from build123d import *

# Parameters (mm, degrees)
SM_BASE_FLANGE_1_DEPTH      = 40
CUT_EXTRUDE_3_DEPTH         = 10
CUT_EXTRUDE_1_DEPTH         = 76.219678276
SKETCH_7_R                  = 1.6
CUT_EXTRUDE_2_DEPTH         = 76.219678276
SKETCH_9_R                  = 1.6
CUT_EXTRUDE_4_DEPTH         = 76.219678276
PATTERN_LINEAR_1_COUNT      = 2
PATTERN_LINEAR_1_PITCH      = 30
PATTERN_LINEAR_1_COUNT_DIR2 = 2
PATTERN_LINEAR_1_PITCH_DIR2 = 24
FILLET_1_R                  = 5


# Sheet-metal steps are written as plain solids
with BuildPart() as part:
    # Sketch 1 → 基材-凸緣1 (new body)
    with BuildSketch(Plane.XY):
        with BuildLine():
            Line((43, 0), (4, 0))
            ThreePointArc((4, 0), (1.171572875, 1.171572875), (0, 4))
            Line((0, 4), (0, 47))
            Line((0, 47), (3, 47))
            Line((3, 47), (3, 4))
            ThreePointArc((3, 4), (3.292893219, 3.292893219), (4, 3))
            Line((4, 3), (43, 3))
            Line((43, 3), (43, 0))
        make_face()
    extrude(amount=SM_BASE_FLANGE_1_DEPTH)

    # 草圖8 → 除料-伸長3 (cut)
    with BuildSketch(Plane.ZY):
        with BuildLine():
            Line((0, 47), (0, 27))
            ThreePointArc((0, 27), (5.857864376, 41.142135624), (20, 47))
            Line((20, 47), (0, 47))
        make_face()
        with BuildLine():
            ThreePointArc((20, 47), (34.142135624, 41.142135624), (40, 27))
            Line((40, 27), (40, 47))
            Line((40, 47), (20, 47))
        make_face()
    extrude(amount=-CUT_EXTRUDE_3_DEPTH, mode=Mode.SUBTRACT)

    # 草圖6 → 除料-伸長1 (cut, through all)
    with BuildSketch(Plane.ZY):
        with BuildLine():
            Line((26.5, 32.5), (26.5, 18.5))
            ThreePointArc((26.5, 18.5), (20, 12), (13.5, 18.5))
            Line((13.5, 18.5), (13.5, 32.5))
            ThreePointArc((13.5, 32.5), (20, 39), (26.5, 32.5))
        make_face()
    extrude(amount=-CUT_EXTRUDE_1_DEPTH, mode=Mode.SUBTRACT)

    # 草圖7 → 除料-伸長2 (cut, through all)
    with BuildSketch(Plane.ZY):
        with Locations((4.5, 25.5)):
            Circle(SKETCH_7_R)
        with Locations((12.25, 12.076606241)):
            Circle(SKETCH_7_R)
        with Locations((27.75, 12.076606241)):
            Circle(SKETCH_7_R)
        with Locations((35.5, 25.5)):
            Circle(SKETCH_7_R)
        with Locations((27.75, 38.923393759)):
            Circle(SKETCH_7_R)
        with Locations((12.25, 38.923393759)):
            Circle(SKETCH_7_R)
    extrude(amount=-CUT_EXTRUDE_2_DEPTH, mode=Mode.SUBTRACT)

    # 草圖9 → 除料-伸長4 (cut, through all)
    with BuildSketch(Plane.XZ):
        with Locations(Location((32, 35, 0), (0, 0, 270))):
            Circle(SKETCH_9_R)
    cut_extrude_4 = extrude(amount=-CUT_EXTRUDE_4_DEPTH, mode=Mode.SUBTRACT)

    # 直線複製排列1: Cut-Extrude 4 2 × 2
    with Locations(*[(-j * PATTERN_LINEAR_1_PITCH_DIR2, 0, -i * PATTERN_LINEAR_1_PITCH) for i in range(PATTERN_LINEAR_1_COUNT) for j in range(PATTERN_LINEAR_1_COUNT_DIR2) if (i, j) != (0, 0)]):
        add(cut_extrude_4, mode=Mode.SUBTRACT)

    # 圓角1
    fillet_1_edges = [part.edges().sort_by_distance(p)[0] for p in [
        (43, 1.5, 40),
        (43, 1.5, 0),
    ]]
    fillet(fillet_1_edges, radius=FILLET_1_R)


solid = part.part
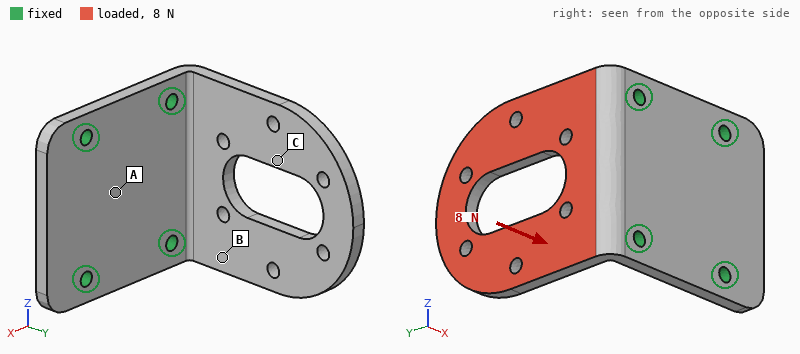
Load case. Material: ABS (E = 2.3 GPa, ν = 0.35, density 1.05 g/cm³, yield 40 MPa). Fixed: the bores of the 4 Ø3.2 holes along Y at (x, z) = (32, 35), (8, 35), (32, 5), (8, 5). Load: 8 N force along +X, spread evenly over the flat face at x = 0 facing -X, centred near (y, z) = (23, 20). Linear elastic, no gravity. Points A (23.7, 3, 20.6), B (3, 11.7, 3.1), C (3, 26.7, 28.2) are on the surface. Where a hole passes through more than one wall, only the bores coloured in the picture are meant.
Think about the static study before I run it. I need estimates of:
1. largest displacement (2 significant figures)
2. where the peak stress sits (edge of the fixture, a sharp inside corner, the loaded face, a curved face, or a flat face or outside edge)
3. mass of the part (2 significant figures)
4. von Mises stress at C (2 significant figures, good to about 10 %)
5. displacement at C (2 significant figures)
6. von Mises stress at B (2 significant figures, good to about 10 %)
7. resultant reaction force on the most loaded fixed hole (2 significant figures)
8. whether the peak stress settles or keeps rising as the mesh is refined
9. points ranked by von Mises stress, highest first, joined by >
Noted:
0.72 mm
edge of the fixture
9.0 g
0.97 MPa
0.32 mm
2.0 MPa
3.0 N
keeps rising
B > C > A
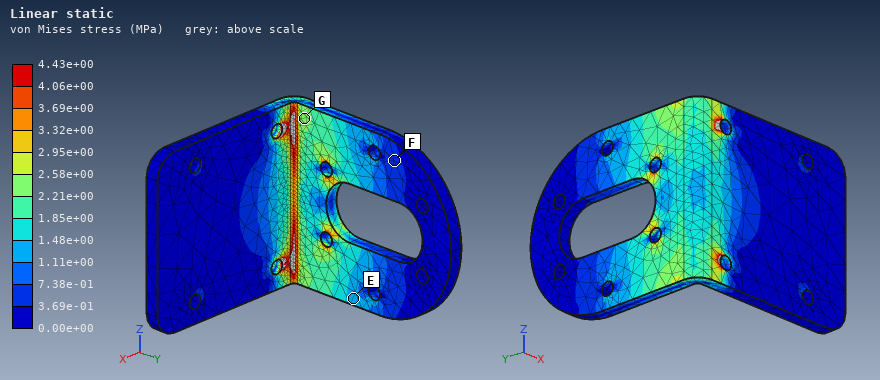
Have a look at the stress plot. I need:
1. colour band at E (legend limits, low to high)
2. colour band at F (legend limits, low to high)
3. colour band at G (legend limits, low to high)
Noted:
1.11e+00 to 1.48e+00 MPa
3.69e-01 to 7.38e-01 MPa
2.21e+00 to 2.58e+00 MPa
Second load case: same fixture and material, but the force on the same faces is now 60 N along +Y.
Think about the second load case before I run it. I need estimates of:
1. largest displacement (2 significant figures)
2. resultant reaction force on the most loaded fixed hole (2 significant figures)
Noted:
0.80 mm
32 N
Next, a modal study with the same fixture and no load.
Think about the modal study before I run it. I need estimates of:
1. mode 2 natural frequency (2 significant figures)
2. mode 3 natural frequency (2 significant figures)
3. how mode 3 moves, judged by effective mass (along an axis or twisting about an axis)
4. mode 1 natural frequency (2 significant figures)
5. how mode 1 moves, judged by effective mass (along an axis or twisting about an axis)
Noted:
920 Hz
1700 Hz
along Z
350 Hz
along X
